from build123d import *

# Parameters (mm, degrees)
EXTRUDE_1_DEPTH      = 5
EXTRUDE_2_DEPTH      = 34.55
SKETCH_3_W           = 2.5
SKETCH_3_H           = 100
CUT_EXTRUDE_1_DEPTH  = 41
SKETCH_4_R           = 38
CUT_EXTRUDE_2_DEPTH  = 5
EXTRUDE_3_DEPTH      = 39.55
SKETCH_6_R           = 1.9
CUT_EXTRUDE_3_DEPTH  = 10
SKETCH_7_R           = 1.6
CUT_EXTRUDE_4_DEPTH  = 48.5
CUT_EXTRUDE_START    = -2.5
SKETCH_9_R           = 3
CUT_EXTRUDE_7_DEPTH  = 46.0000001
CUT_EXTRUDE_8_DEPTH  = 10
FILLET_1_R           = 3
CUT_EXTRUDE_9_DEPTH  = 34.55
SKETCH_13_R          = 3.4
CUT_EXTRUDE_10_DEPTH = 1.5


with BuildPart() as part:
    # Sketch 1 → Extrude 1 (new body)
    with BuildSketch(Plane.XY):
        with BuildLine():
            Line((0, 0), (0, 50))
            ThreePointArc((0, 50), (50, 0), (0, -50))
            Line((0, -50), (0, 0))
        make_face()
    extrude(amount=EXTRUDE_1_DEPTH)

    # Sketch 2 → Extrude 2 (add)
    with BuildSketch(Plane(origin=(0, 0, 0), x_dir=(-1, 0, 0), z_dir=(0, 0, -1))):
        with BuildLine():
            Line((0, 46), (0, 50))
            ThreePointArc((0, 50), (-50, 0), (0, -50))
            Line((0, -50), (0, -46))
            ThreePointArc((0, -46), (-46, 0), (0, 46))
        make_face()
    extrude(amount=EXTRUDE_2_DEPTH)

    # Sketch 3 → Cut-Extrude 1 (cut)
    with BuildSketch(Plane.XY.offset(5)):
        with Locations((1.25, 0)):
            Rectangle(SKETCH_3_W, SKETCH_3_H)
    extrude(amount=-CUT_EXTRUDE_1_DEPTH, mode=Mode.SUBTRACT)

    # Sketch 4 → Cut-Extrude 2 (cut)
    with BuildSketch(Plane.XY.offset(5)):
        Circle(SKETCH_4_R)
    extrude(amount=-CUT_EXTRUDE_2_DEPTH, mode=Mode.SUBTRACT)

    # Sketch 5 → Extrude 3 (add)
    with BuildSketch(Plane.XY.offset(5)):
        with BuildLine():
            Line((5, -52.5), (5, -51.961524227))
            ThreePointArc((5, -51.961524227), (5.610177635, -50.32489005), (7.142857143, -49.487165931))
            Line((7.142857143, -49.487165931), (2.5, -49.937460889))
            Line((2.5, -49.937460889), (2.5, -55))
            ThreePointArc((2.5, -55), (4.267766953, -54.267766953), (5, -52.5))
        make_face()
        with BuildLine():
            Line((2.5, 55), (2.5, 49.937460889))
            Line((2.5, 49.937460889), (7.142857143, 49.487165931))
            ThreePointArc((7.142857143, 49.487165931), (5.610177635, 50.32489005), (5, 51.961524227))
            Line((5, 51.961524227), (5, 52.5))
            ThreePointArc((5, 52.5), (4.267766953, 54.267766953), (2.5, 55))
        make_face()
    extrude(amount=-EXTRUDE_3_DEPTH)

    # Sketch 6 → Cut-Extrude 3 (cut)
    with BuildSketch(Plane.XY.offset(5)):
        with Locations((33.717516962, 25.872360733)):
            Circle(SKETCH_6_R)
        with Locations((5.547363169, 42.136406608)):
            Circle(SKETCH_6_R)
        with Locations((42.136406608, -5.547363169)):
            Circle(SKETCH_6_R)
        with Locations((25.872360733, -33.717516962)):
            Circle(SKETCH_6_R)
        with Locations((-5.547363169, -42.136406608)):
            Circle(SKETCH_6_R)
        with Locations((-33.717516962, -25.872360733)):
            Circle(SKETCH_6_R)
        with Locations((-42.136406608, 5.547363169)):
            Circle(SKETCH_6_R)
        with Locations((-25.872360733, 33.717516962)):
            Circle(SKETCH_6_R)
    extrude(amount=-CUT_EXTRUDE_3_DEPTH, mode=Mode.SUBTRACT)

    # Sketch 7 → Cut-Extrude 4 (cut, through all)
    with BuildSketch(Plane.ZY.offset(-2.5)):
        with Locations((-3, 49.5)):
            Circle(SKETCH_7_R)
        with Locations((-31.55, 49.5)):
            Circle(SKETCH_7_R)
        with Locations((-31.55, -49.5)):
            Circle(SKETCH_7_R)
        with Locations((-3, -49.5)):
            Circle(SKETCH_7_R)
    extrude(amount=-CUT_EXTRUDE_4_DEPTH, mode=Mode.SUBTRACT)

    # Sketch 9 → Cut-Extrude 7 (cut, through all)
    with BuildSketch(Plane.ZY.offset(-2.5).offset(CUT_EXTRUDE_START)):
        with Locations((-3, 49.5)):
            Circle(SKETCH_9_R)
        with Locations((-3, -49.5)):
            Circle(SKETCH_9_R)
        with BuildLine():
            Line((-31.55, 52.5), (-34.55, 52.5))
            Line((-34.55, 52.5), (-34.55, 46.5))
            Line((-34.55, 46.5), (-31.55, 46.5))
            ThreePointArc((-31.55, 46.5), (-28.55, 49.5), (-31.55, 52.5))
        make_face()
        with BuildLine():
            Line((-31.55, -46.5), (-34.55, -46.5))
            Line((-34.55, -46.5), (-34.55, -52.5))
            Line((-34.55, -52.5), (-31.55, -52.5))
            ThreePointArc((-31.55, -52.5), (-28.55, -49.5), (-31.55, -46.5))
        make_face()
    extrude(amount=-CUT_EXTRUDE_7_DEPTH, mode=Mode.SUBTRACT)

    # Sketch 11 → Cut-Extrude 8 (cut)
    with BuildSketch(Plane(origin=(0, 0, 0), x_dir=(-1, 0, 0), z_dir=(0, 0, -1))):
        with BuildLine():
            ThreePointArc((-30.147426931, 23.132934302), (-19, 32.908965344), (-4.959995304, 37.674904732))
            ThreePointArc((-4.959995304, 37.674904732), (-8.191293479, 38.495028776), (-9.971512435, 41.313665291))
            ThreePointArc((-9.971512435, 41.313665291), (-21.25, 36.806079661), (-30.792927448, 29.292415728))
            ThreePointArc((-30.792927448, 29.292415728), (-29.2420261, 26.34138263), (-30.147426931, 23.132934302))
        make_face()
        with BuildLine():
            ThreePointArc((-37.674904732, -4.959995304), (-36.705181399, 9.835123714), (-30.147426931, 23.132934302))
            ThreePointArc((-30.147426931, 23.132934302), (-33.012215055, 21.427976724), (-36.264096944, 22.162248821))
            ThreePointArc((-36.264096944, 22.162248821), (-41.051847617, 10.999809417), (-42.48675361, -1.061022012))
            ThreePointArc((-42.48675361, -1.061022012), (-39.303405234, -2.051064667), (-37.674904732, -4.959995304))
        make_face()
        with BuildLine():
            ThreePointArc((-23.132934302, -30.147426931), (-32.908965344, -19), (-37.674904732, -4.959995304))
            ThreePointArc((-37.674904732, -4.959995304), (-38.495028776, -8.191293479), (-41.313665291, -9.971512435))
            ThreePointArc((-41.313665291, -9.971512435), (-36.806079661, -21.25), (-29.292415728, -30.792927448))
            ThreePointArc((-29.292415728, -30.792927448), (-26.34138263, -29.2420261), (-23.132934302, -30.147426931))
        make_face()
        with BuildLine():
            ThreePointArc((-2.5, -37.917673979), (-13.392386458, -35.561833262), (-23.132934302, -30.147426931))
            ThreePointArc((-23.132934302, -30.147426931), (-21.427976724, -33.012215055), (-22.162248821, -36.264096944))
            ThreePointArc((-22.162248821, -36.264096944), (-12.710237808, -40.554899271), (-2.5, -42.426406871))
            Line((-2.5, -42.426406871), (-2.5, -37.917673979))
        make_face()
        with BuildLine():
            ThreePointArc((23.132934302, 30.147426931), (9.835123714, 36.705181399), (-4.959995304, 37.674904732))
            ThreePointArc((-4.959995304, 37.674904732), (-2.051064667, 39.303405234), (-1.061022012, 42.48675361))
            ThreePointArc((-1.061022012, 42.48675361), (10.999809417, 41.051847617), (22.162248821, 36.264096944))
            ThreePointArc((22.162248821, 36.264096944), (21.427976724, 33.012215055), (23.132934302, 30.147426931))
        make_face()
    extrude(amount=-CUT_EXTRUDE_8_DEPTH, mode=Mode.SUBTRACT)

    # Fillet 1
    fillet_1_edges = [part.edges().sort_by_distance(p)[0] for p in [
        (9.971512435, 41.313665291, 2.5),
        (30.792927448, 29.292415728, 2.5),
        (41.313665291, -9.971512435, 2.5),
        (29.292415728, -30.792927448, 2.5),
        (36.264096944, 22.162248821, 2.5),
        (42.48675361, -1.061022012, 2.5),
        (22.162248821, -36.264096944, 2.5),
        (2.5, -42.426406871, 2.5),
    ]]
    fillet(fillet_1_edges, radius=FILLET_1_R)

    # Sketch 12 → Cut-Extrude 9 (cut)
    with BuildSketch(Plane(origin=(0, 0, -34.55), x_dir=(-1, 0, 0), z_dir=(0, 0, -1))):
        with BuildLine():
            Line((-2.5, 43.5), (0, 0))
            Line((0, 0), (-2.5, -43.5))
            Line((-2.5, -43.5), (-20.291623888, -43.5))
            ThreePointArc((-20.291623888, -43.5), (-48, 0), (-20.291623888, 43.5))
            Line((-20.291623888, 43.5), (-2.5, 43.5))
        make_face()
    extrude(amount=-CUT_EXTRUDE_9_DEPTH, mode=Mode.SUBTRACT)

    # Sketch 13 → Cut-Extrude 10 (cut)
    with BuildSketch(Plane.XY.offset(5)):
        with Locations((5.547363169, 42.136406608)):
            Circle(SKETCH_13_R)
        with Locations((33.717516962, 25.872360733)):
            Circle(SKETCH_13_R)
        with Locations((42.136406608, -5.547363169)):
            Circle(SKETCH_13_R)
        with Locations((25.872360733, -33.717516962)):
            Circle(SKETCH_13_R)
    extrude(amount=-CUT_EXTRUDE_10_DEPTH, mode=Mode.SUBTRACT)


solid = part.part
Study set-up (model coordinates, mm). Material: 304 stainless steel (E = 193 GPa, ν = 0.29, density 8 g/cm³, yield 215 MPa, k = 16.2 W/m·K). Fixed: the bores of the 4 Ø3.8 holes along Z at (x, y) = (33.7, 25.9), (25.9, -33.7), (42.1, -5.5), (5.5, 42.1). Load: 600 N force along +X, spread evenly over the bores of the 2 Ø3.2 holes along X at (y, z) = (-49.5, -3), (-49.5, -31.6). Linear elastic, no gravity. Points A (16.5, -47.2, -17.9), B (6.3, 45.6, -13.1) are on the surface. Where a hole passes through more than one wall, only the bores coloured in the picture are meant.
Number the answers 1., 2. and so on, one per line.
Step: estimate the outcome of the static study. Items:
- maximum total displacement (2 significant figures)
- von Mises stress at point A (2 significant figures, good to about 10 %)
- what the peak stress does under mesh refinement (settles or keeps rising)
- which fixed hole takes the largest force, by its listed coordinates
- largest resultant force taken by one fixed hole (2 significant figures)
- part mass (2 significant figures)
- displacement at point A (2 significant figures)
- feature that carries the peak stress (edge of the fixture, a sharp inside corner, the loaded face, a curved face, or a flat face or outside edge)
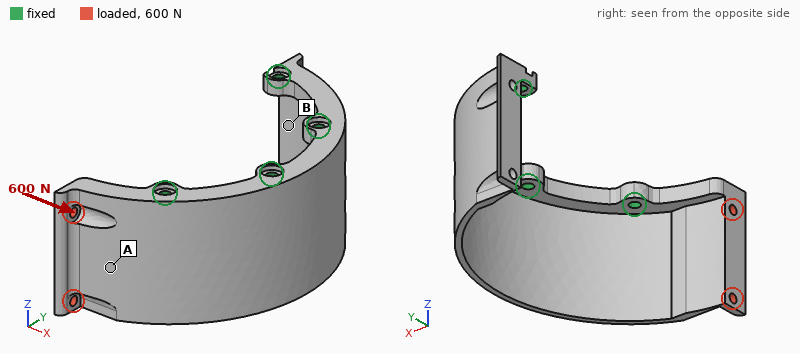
1. 0.24 mm
2. 29 MPa
3. keeps rising
4. (25.9, -33.7)
5. 690 N
6. 150 g
7. 0.11 mm
8. edge of the fixture
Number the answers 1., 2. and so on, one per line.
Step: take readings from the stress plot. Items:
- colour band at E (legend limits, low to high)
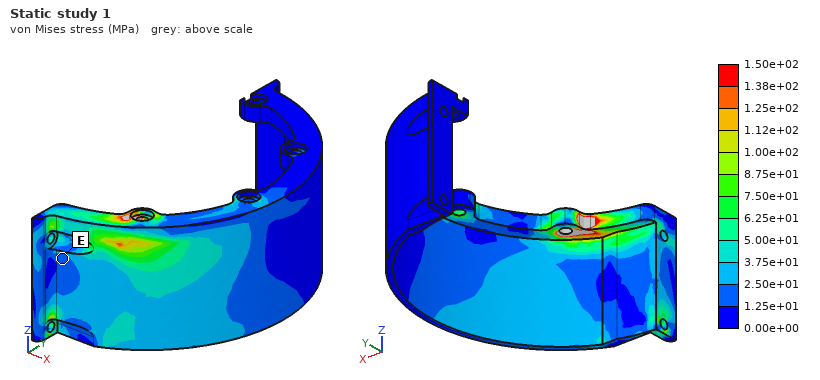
1. 1.25e+01 to 2.50e+01 MPa
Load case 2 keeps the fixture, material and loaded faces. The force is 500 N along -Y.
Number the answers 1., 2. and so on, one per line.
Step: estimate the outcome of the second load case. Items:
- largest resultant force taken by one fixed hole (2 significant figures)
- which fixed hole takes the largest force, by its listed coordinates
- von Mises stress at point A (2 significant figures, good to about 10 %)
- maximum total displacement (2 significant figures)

1. 970 N
2. (25.9, -33.7)
3. 89 MPa
4. 0.37 mm
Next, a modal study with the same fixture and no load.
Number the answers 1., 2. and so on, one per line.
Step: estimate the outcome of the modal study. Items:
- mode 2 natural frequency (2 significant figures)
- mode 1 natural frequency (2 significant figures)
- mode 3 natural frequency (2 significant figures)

1. 2500 Hz
2. 1600 Hz
3. 2600 Hz
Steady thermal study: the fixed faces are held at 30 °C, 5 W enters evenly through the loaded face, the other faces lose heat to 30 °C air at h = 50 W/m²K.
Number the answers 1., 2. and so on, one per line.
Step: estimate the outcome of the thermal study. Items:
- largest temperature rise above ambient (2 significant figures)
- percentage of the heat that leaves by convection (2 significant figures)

1. 72 K
2. 83 %
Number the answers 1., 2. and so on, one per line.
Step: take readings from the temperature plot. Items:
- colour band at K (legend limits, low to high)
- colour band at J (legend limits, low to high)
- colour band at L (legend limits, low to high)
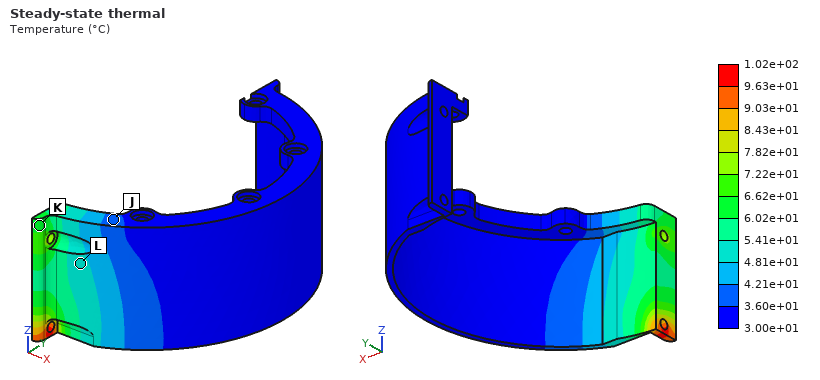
1. 6.02e+01 to 6.62e+01 °C
2. 3.60e+01 to 4.21e+01 °C
3. 4.81e+01 to 5.41e+01 °C
